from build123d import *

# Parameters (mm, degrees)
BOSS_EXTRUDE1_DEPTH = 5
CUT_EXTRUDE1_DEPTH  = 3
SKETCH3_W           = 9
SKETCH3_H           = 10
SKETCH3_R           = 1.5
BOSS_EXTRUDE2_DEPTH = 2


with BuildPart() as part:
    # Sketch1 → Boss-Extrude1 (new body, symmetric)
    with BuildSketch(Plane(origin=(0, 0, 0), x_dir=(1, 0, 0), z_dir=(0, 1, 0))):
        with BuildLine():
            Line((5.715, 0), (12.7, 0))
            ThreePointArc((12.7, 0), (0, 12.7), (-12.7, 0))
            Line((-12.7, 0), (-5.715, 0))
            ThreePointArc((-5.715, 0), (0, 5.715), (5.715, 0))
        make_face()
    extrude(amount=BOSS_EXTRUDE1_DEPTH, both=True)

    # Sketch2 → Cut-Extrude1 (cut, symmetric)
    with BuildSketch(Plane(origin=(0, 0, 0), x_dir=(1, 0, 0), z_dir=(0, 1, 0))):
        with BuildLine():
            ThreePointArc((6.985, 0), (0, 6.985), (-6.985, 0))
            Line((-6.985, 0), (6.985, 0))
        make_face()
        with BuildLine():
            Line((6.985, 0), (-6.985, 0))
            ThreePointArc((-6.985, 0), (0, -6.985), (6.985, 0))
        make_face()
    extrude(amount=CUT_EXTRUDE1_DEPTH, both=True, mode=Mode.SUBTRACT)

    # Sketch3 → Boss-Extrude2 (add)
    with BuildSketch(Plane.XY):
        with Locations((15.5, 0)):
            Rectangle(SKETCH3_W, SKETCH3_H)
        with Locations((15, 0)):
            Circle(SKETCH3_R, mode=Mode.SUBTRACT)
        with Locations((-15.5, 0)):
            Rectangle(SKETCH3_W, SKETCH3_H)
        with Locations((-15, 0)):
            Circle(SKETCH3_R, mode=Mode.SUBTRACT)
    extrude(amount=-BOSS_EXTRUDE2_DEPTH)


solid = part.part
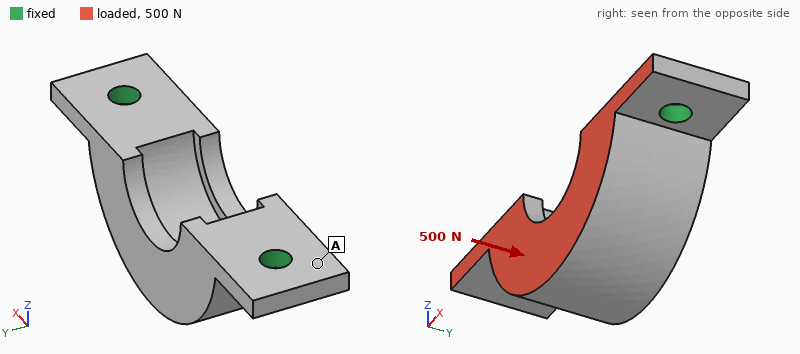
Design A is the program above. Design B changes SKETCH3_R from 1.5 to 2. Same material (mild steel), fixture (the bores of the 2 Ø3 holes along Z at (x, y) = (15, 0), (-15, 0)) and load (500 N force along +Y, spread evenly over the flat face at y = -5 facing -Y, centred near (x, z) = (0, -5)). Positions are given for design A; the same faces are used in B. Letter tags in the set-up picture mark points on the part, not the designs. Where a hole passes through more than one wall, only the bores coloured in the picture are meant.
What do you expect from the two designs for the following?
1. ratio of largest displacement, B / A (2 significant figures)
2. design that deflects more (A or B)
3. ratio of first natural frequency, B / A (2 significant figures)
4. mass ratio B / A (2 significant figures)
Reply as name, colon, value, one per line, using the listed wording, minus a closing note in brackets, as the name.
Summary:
ratio of largest displacement, B / A: 0.70
design that deflects more: A
ratio of first natural frequency, B / A: 1.2
mass ratio B / A: 0.99
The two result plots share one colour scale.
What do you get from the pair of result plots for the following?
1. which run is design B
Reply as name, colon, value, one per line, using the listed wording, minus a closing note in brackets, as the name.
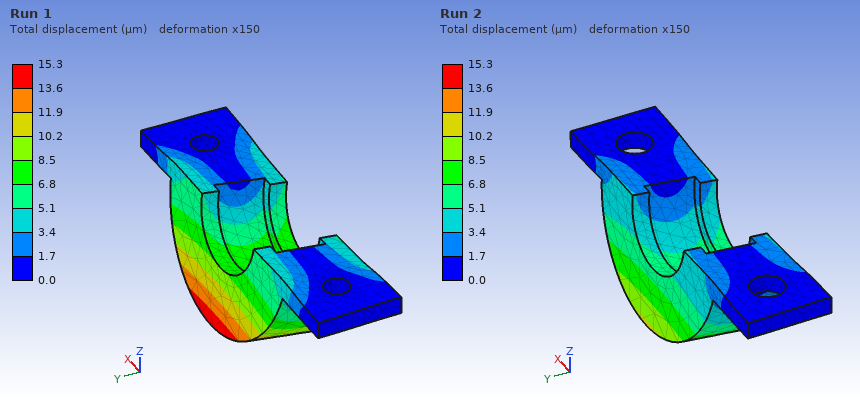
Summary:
which run is design B: Run 2
